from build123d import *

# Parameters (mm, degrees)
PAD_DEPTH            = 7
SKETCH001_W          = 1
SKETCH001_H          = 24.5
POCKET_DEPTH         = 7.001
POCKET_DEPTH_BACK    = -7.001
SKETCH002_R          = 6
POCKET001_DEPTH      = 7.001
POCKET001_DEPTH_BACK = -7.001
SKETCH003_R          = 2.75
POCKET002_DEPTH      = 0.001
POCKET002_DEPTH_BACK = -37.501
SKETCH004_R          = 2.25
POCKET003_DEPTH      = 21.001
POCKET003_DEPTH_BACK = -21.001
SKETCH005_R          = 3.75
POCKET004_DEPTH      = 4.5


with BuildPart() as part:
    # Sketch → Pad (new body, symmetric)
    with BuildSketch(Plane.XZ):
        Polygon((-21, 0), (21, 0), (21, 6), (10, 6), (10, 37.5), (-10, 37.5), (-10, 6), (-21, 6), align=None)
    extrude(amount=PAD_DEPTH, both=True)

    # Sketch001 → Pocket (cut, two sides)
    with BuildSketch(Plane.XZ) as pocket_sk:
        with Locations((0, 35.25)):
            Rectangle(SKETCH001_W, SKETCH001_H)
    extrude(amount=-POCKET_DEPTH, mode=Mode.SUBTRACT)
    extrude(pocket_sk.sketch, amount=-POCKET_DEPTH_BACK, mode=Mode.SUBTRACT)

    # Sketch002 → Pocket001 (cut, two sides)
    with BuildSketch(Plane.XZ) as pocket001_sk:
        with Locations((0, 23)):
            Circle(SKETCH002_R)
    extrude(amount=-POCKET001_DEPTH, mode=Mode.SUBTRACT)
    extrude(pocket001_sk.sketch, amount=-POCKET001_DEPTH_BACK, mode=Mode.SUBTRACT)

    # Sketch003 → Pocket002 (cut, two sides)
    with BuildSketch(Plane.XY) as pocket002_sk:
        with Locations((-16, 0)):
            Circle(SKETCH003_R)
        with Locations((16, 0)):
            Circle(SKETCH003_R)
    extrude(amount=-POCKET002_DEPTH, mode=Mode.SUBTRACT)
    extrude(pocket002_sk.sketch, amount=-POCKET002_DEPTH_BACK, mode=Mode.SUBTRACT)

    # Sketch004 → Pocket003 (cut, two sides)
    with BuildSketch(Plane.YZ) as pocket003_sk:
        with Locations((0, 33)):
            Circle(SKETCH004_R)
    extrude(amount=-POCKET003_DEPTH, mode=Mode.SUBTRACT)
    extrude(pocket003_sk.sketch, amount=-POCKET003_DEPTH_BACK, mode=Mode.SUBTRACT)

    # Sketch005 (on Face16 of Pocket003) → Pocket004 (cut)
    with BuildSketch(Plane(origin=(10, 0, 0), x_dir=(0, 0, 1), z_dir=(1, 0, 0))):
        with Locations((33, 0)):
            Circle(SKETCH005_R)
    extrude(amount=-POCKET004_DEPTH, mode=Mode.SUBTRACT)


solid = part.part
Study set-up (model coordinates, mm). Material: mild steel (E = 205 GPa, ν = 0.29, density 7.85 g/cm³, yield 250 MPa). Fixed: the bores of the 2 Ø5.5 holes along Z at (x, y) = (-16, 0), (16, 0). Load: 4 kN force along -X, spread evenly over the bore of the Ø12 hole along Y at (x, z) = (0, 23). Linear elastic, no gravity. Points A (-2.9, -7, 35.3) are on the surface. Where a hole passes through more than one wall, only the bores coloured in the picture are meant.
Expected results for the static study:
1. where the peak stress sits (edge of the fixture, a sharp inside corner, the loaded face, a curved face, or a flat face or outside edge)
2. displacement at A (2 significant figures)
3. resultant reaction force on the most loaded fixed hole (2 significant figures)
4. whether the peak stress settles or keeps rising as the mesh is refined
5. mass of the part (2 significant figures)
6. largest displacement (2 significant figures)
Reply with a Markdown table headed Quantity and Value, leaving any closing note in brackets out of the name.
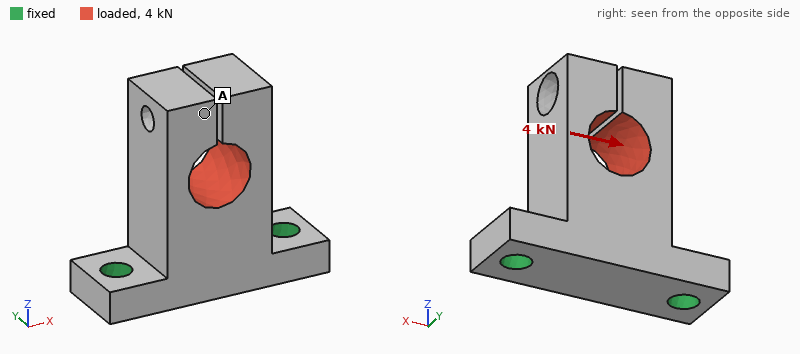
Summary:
| Quantity | Value |
|---|---|
| where the peak stress sits | edge of the fixture |
| displacement at A | 64 µm |
| resultant reaction force on the most loaded fixed hole | 3.8 kN |
| whether the peak stress settles or keeps rising as the mesh is refined | keeps rising |
| mass of the part | 78 g |
| largest displacement | 73 µm |
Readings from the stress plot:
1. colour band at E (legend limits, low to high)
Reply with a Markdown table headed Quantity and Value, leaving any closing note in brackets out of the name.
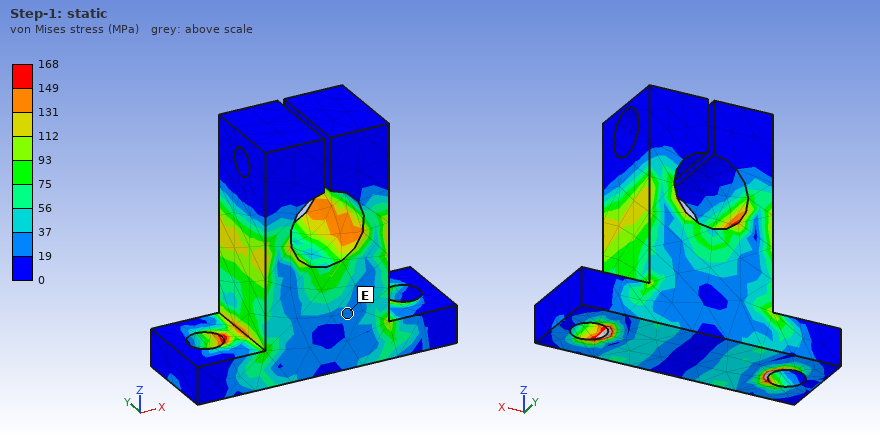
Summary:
| Quantity | Value |
|---|---|
| colour band at E | 19 to 37 MPa |
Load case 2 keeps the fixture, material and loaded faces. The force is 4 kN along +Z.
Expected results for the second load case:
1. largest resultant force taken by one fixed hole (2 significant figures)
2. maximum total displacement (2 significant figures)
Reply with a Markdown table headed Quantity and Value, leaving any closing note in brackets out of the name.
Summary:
| Quantity | Value |
|---|---|
| largest resultant force taken by one fixed hole | 2.1 kN |
| maximum total displacement | 37 µm |
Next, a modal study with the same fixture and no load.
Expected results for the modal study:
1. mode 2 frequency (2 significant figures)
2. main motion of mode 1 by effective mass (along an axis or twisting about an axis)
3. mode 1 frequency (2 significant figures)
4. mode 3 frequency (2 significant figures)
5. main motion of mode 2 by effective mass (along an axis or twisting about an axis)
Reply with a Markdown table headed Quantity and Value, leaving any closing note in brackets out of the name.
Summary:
| Quantity | Value |
|---|---|
| mode 2 frequency | 5600 Hz |
| main motion of mode 1 by effective mass | along Y |
| mode 1 frequency | 4500 Hz |
| mode 3 frequency | 6100 Hz |
| main motion of mode 2 by effective mass | along X |
